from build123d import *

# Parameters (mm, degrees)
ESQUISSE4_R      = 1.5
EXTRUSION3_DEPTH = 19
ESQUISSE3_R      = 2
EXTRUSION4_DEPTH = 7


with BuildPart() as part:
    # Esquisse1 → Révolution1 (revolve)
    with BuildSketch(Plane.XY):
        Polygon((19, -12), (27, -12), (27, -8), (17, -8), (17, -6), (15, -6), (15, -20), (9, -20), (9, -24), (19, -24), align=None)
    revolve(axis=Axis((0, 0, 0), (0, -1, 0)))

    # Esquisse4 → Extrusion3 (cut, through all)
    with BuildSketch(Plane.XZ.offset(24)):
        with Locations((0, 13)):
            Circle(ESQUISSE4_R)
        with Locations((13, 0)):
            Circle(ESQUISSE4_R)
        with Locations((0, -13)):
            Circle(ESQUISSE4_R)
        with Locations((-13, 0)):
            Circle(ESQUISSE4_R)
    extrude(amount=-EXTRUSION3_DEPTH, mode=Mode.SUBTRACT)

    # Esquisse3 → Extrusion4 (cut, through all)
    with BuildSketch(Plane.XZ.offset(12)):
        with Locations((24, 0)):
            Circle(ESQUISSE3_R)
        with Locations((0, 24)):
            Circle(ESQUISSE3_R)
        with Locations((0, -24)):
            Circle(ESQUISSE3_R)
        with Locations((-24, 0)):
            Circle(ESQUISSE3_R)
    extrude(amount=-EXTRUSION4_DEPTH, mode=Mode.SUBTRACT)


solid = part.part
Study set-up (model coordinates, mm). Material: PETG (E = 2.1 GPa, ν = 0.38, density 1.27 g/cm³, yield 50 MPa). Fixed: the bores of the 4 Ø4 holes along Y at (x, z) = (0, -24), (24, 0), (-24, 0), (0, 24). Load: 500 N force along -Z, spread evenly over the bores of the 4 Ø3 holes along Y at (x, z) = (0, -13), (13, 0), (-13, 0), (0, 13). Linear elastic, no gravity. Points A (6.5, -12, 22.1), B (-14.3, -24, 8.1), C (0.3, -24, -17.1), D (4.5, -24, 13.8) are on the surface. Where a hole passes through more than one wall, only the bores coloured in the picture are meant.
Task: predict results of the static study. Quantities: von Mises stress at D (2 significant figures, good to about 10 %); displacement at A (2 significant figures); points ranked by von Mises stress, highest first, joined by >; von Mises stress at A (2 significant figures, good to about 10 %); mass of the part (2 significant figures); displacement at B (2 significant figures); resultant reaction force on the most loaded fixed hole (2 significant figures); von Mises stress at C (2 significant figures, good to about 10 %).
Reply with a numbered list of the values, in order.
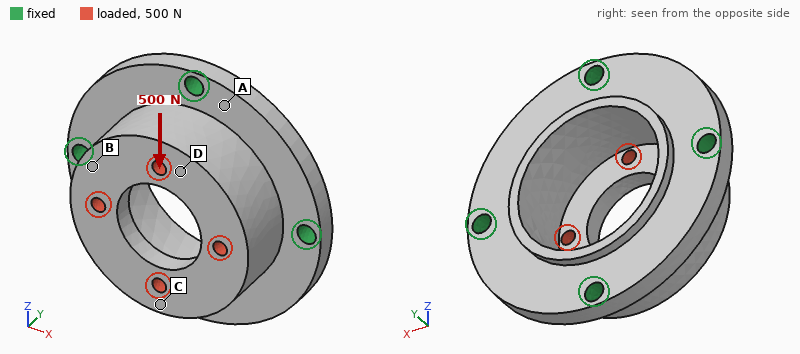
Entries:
1. 3.8 MPa
2. 0.022 mm
3. C > D > A > B
4. 2.2 MPa
5. 17 g
6. 0.071 mm
7. 180 N
8. 5.2 MPa
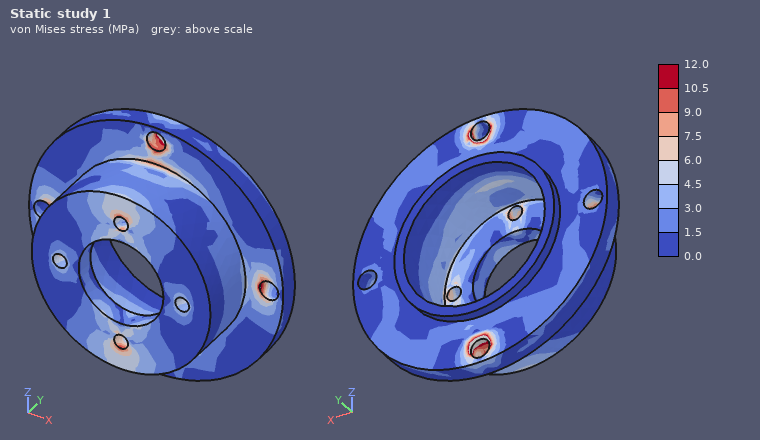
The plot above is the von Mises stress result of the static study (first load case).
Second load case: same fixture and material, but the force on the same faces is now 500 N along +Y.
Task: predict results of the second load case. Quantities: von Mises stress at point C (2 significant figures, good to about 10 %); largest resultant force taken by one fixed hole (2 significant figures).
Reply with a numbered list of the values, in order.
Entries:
1. 3.3 MPa
2. 140 N
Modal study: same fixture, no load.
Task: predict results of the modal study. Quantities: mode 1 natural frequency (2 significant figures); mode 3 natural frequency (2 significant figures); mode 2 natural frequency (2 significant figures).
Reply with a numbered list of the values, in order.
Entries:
1. 4200 Hz
2. 4300 Hz
3. 4200 Hz
